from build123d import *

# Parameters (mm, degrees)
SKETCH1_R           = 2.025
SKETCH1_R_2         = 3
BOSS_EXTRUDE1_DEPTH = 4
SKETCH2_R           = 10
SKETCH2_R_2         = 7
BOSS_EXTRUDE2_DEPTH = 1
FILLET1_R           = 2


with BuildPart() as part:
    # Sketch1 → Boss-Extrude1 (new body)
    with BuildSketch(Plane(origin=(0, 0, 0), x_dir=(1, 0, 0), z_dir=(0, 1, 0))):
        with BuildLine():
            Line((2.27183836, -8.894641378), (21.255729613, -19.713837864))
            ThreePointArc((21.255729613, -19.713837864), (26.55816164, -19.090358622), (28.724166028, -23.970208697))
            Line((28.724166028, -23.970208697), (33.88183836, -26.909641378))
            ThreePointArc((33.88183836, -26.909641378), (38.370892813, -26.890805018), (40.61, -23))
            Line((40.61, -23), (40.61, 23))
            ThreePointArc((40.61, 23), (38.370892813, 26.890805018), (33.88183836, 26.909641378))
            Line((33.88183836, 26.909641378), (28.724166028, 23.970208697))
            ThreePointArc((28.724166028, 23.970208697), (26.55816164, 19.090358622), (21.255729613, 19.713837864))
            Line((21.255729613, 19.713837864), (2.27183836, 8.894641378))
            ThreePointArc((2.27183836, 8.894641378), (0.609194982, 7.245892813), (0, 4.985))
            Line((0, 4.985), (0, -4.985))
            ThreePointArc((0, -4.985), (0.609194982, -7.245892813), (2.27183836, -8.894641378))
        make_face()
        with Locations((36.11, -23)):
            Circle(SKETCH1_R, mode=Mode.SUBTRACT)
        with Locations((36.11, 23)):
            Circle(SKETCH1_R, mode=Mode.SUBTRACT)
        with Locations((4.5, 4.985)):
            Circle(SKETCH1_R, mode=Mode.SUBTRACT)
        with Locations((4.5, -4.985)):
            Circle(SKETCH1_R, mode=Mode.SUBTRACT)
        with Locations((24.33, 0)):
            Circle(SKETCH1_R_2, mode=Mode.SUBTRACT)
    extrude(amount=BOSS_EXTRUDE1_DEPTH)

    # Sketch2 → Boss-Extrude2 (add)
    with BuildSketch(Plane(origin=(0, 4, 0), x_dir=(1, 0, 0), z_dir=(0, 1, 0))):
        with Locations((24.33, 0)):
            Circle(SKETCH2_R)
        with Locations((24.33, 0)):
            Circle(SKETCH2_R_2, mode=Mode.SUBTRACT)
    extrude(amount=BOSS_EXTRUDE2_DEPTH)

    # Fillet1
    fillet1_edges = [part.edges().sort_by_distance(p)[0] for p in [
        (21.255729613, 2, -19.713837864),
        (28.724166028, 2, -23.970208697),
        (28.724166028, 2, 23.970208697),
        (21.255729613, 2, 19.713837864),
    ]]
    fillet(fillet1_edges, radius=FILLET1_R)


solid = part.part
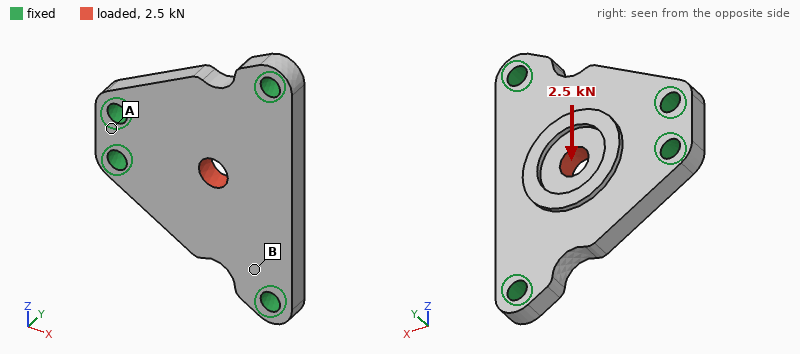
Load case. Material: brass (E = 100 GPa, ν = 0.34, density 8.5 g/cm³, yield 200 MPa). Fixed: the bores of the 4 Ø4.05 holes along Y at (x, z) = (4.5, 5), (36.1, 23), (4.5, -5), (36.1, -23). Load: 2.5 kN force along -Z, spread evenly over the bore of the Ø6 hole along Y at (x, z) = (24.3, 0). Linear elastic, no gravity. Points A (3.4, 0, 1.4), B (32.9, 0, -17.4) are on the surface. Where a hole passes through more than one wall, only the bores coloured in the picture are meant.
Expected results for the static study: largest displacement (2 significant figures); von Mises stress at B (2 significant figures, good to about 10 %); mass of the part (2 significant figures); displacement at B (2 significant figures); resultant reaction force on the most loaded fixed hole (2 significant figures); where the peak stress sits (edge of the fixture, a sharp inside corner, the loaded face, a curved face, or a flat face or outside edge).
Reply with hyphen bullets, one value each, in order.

- 5.9 µm
- 22 MPa
- 49 g
- 1.5 µm
- 910 N
- the loaded face
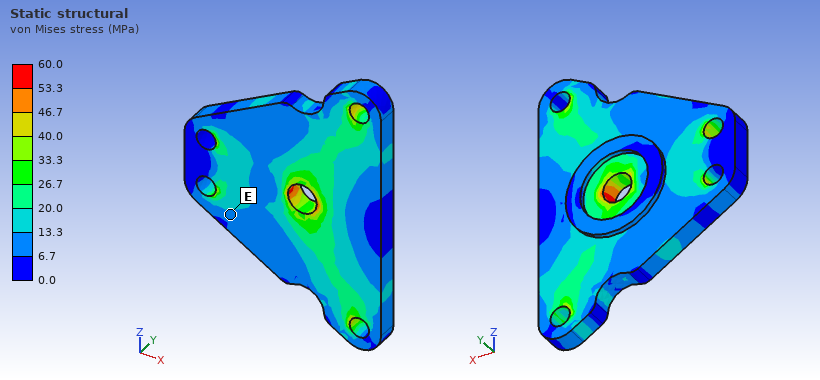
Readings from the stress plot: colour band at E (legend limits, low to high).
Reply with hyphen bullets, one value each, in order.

- 6.7 to 13.3 MPa
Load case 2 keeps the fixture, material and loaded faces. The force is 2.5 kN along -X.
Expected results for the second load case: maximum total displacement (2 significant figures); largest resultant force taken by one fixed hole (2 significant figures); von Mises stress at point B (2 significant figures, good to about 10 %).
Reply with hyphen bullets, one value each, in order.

- 6.9 µm
- 940 N
- 12 MPa
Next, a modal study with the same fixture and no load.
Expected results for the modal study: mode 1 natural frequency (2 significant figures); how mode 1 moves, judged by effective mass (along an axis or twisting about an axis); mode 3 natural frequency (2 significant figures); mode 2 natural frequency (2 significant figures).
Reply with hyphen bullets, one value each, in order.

- 7100 Hz
- along Y
- 12 kHz
- 12 kHz
